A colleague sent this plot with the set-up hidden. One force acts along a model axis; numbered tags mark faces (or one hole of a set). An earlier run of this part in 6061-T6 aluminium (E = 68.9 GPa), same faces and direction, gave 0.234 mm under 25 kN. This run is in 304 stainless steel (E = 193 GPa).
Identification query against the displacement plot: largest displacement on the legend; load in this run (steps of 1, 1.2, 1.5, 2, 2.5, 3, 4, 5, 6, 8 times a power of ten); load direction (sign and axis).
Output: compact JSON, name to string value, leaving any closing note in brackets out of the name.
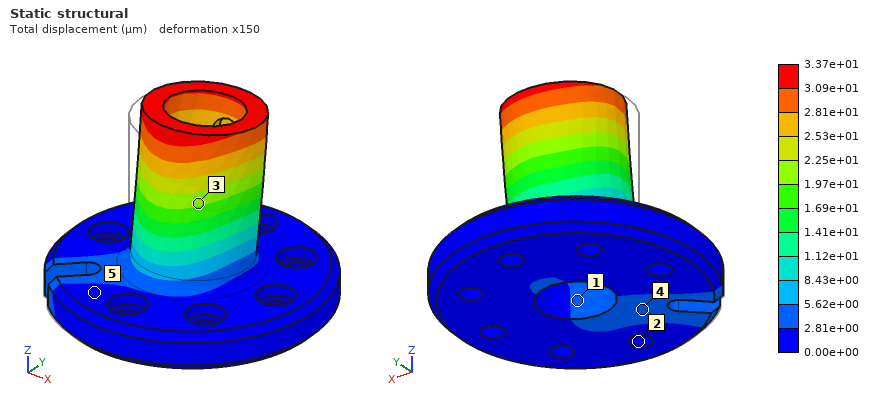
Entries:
{"largest displacement on the legend": "3.37e+01 µm", "load in this run": "10 kN", "load direction": "+Y"}
